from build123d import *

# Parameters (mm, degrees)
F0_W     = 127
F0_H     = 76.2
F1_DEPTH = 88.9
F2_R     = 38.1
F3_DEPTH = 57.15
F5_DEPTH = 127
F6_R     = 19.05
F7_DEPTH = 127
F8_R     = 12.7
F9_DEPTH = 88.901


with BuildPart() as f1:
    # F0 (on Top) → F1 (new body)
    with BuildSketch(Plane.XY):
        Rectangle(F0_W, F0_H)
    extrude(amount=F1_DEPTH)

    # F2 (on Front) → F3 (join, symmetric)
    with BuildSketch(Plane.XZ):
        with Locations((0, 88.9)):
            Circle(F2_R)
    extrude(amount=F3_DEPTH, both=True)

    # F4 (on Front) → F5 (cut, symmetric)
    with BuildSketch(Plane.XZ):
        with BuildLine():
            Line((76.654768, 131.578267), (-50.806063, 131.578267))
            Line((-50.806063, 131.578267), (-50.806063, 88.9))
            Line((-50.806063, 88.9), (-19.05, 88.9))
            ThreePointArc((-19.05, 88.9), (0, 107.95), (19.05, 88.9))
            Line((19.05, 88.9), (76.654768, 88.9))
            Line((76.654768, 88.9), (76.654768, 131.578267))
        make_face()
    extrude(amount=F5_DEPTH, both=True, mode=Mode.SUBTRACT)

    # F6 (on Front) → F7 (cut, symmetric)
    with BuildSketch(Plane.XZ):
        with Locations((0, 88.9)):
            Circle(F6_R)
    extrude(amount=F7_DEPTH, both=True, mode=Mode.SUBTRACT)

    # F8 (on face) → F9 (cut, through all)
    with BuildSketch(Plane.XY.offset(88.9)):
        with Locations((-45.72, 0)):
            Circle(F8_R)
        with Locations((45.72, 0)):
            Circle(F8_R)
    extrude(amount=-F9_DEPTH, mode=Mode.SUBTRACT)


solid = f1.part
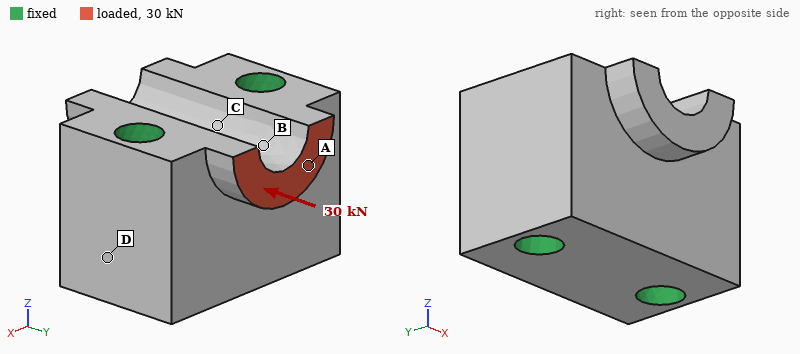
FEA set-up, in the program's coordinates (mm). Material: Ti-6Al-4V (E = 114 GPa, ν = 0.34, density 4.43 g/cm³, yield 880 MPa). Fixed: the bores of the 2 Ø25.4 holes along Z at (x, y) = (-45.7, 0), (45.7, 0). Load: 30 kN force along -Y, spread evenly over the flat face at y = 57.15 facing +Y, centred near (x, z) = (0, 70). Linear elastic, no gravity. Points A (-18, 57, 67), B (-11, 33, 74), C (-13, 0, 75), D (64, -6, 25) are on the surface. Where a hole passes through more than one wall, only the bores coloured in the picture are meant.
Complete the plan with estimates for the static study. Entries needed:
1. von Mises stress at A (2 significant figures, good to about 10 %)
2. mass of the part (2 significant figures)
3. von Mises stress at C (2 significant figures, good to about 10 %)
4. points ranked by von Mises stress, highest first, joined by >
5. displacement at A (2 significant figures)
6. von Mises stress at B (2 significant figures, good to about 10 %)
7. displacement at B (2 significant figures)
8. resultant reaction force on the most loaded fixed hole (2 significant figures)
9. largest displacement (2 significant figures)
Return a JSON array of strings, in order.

["17 MPa", "3.5 kg", "5.4 MPa", "A > B > C > D", "7.2 µm", "12 MPa", "4.7 µm", "16 kN", "10 µm"]
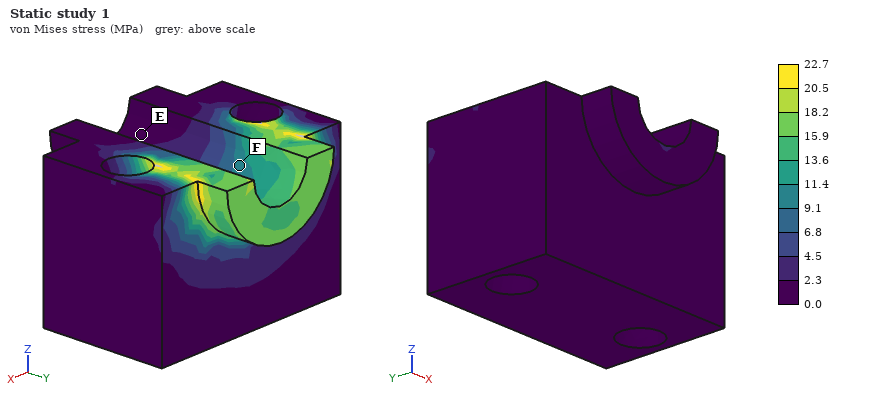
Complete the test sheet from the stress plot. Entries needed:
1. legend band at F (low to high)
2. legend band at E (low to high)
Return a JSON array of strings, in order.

["9.1 to 11.4 MPa", "0.0 to 2.3 MPa"]
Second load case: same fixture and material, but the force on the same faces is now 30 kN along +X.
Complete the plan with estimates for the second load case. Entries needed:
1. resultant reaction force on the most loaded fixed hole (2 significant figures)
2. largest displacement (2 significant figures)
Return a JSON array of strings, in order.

["22 kN", "37 µm"]
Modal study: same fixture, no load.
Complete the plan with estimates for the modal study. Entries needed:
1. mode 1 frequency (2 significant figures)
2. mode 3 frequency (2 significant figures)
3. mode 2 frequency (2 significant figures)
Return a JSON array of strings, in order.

["14 kHz", "15 kHz", "14 kHz"]
